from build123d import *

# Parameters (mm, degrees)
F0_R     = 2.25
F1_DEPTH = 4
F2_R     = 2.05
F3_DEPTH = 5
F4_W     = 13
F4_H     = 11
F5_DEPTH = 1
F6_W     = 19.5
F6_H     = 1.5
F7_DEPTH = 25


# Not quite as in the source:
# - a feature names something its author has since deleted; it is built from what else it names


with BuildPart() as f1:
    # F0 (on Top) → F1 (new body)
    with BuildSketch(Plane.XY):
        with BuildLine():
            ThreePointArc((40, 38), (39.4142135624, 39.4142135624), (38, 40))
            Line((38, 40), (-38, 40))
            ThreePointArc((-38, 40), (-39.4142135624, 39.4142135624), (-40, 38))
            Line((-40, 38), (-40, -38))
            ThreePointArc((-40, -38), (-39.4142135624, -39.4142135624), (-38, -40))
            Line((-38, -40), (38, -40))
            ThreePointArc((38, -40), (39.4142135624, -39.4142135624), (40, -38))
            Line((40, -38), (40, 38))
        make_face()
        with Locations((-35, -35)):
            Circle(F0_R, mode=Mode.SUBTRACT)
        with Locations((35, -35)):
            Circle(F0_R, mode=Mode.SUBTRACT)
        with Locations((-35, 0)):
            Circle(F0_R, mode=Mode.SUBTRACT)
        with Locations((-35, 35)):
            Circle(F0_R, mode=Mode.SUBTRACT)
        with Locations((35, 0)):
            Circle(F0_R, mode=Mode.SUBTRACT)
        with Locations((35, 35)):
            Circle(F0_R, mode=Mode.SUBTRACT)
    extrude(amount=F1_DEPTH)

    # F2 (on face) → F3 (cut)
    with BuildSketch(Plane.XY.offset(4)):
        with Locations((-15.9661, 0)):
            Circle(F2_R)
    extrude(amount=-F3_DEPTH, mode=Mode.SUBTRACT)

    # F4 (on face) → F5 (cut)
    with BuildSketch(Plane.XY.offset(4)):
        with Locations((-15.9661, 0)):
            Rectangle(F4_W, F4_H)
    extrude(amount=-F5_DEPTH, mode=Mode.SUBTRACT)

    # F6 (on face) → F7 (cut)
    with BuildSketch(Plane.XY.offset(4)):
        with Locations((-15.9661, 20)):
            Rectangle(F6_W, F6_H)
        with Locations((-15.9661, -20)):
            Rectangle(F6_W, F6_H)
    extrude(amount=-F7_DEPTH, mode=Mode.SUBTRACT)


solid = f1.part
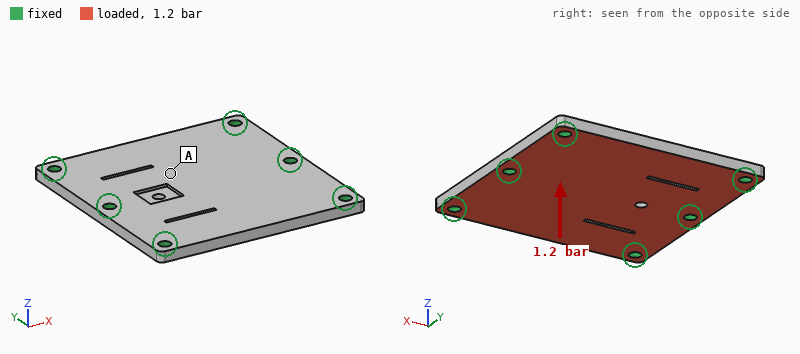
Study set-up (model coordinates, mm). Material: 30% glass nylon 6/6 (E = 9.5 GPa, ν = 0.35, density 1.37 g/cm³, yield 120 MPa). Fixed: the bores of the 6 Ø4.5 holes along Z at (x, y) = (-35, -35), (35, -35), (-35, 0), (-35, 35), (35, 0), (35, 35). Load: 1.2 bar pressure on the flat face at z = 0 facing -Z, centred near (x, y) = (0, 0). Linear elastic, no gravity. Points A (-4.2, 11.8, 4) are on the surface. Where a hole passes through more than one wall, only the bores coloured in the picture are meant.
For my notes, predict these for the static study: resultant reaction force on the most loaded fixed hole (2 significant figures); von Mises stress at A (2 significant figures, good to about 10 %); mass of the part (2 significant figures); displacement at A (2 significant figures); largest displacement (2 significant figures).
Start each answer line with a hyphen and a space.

- 170 N
- 8.5 MPa
- 34 g
- 0.17 mm
- 0.17 mm
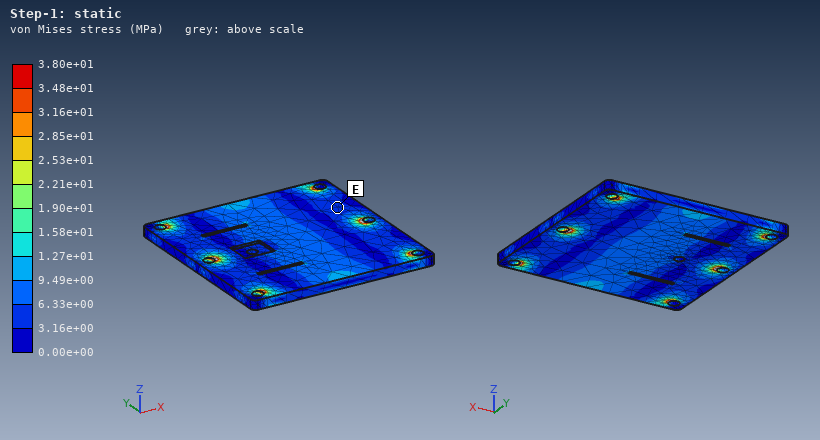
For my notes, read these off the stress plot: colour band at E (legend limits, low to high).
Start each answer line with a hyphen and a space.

- 3.16e+00 to 6.33e+00 MPa
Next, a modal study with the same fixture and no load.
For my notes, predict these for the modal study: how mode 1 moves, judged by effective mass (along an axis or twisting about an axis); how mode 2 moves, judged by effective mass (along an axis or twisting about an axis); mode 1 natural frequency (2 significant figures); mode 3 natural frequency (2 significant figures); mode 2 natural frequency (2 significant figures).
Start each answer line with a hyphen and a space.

- along Z
- twisting about X
- 2000 Hz
- 3700 Hz
- 2400 Hz
